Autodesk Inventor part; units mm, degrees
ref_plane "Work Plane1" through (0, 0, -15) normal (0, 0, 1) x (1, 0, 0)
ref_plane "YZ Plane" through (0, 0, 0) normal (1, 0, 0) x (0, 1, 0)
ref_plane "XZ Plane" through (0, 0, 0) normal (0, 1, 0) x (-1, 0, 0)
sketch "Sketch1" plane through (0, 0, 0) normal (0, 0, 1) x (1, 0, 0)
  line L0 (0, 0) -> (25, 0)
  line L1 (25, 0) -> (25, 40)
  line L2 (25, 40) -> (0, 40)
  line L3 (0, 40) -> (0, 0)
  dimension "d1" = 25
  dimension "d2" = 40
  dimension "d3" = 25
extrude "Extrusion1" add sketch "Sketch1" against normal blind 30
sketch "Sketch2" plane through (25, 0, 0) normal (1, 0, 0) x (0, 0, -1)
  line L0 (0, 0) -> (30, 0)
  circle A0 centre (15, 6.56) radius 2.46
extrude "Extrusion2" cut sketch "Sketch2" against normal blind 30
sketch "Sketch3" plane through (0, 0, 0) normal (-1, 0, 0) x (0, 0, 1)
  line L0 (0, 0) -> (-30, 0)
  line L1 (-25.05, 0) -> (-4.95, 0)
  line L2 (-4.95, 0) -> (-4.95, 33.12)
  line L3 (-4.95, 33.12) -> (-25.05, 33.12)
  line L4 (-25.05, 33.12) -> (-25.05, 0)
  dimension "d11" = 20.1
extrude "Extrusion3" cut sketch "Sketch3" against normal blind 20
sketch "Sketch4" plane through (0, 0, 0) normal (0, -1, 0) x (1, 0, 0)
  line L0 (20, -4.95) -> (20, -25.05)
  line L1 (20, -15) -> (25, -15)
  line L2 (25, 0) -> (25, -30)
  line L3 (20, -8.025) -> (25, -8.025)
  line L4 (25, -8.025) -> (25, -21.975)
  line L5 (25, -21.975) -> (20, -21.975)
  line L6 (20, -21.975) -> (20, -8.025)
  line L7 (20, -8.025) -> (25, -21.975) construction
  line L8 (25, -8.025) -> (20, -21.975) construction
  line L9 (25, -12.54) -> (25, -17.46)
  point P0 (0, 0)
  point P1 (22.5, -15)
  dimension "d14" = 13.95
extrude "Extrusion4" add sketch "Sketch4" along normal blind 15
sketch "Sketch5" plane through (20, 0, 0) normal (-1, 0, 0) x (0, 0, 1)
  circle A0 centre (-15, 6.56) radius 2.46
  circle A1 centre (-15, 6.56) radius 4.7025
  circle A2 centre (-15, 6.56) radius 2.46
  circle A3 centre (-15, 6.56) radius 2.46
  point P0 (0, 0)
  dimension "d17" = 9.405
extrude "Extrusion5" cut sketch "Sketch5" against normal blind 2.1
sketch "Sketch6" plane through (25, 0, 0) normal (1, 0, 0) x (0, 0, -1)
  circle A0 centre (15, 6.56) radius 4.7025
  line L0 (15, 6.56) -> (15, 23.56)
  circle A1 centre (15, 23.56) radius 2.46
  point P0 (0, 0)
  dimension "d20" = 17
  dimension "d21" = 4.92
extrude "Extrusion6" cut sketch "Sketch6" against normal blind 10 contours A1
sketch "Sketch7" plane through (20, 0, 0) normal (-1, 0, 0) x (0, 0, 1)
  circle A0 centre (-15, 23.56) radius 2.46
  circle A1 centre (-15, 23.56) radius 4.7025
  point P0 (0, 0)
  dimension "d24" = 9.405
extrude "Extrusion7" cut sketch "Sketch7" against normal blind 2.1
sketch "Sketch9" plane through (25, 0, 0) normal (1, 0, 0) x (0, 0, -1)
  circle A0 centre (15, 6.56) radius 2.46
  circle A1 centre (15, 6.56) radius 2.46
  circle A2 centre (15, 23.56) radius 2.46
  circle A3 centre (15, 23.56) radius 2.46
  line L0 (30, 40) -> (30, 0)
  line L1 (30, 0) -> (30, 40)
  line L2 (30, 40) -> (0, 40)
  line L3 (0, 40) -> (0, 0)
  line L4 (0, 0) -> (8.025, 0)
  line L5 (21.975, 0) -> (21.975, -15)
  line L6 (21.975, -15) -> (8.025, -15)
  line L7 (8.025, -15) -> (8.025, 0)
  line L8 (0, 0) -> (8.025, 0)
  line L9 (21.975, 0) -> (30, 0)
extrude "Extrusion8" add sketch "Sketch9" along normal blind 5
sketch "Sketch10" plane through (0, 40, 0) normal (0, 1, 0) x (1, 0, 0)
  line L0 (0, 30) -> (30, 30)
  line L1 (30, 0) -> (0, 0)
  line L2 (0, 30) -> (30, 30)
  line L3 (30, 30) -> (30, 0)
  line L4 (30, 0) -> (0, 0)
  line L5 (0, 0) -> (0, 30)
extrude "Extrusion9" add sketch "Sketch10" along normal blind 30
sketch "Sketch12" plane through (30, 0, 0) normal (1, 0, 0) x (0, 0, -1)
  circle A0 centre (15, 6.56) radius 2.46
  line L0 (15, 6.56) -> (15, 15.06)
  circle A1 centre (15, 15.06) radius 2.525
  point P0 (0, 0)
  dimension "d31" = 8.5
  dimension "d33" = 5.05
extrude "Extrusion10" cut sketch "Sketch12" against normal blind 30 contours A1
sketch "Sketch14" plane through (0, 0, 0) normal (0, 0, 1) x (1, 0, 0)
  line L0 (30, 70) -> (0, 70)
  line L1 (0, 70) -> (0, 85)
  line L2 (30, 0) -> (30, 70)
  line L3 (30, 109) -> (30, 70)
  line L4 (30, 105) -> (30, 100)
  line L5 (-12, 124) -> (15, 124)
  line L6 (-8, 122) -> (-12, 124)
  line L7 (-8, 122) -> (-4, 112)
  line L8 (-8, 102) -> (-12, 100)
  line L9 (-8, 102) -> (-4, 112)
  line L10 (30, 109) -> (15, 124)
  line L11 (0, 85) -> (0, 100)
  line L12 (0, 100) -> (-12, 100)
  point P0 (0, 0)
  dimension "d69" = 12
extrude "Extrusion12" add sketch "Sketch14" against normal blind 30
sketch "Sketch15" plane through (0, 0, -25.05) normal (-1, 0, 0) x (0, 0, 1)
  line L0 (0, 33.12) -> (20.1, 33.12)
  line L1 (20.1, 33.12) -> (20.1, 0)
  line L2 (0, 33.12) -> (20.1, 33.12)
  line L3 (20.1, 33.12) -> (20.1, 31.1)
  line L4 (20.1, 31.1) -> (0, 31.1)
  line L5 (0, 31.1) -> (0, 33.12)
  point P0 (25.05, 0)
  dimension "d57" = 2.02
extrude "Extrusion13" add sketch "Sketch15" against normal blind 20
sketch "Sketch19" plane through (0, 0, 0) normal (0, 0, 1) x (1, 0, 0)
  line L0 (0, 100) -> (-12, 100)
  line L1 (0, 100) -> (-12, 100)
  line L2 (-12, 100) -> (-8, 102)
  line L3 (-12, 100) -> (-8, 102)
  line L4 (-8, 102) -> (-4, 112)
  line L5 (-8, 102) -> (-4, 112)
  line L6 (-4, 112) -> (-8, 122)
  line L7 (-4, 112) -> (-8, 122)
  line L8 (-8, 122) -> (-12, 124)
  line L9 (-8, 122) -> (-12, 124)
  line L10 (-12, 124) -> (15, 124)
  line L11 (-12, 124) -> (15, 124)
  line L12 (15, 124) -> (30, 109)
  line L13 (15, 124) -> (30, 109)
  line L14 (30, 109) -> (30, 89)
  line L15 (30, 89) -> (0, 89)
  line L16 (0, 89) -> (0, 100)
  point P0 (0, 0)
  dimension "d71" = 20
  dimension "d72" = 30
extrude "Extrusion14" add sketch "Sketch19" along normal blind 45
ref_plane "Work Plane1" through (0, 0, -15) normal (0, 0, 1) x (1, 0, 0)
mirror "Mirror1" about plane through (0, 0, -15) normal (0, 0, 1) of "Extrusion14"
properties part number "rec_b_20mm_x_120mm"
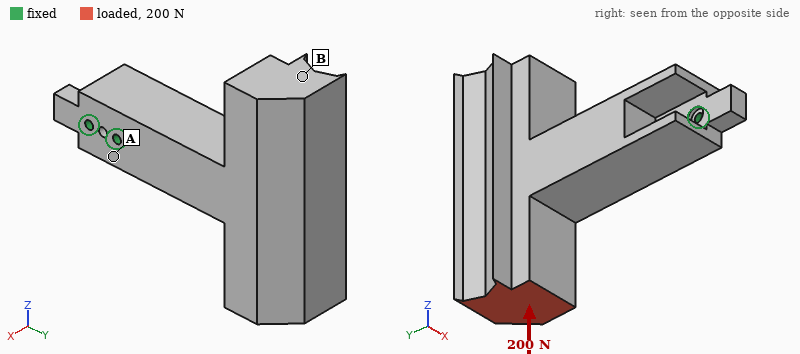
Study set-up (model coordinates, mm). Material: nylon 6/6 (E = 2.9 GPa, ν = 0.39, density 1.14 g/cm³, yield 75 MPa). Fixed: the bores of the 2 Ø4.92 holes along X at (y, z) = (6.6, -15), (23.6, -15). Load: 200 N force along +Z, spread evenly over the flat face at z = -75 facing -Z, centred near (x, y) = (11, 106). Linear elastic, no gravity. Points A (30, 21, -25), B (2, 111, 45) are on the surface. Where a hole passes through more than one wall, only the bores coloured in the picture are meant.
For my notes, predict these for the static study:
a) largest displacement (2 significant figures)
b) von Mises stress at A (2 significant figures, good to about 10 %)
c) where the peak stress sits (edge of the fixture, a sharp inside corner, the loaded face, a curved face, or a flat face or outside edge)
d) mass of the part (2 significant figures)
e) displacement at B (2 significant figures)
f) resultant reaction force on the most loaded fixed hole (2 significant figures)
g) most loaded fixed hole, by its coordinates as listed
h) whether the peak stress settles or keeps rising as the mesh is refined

1.0 mm
5.5 MPa
edge of the fixture
230 g
0.90 mm
920 N
(23.6, -15)
keeps rising
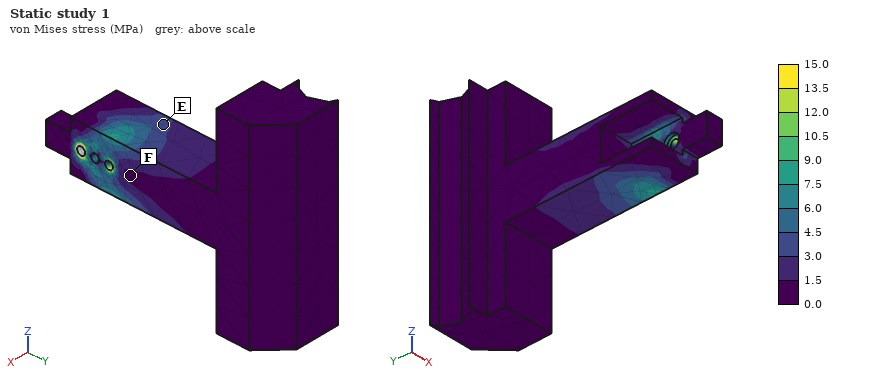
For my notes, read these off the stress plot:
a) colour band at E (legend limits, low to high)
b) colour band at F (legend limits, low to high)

3.0 to 4.5 MPa
0.0 to 1.5 MPa
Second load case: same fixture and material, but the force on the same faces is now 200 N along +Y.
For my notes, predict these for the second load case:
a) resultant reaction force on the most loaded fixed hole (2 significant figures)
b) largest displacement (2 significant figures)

550 N
0.97 mm
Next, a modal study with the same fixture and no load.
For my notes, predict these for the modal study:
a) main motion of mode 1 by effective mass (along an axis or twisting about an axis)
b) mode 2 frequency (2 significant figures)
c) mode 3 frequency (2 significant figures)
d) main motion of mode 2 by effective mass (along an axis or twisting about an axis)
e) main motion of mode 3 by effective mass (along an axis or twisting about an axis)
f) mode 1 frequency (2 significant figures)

along X
200 Hz
270 Hz
along Z
twisting about Y
180 Hz
